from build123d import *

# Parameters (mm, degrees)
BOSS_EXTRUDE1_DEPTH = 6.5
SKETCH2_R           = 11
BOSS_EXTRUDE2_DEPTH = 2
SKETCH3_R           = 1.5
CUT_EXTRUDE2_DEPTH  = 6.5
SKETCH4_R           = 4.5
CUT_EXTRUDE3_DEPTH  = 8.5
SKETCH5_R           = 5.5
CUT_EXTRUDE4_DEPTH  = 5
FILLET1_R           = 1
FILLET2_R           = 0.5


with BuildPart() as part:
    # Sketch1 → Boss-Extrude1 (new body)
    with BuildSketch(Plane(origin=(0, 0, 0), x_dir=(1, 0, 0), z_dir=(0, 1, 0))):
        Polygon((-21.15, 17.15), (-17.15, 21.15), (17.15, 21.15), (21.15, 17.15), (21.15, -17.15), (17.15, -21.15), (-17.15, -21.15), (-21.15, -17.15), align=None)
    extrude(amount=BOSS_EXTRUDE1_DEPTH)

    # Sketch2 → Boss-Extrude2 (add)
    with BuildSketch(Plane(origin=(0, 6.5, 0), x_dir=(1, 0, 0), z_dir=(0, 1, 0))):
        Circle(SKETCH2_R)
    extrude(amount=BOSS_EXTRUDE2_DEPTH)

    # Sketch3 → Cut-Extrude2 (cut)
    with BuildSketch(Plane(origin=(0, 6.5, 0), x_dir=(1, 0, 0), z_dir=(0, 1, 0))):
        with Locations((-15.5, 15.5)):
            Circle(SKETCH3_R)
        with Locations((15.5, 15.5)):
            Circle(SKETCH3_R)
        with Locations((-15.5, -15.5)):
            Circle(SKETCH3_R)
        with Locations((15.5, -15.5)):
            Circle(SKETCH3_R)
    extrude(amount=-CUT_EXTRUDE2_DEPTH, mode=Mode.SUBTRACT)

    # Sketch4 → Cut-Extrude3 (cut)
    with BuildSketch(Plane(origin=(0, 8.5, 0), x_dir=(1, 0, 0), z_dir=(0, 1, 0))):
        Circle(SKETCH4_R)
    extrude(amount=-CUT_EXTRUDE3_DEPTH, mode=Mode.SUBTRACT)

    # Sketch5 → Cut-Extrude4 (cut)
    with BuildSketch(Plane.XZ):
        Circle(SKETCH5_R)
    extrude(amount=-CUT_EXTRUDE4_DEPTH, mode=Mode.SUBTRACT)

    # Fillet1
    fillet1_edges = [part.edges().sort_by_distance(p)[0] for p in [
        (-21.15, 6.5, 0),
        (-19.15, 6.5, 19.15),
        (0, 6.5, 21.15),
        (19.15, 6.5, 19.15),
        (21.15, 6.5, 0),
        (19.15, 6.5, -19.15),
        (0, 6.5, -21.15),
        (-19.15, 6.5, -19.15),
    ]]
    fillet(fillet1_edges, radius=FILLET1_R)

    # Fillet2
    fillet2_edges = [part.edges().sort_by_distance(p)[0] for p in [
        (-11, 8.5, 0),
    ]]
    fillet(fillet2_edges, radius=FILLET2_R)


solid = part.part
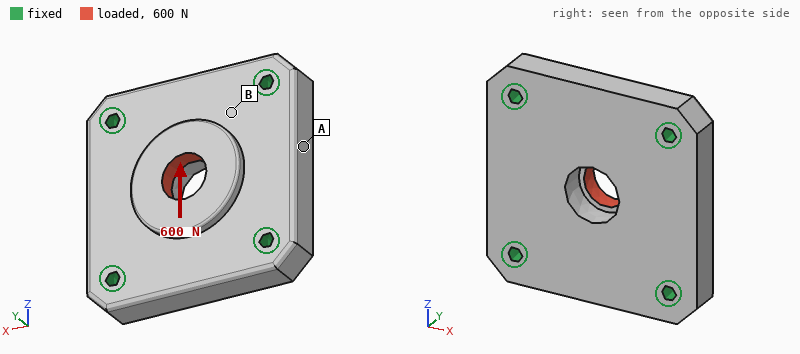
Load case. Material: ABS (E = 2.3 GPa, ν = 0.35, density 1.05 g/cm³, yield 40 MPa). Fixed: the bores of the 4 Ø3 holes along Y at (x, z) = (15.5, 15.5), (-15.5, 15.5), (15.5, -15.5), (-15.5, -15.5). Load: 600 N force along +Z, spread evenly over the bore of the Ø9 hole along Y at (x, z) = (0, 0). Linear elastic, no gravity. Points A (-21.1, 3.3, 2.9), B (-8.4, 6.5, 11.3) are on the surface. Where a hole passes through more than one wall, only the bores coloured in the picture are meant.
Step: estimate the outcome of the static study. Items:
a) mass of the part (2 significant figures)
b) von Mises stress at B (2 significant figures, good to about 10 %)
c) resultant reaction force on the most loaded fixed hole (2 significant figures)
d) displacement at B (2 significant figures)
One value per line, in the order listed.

12 g
3.6 MPa
170 N
15 µm
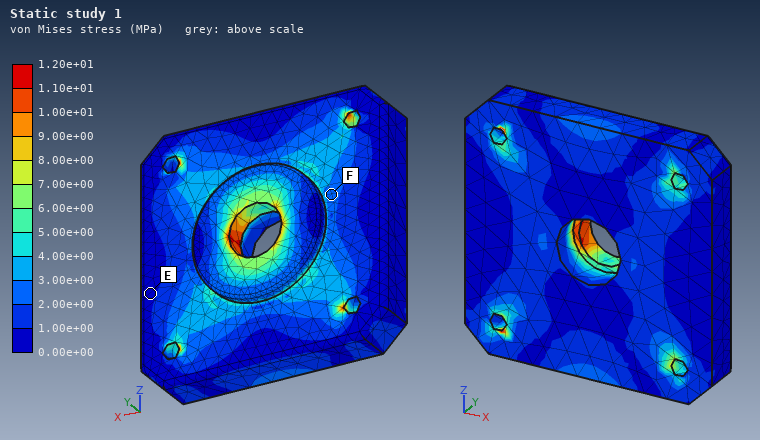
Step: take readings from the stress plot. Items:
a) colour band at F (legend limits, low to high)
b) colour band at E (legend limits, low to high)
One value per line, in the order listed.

2.00e+00 to 3.00e+00 MPa
0.00e+00 to 1.00e+00 MPa
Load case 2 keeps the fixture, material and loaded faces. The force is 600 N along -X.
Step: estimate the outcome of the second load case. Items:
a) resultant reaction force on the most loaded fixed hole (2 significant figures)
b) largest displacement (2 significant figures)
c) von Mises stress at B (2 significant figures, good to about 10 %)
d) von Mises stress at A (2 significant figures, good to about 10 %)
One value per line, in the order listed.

170 N
45 µm
3.4 MPa
1.8 MPa
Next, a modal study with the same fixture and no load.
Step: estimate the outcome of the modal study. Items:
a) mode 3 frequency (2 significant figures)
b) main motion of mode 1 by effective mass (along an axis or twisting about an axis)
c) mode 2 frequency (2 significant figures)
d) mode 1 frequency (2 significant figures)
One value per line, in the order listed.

8500 Hz
along Y
8500 Hz
6000 Hz
